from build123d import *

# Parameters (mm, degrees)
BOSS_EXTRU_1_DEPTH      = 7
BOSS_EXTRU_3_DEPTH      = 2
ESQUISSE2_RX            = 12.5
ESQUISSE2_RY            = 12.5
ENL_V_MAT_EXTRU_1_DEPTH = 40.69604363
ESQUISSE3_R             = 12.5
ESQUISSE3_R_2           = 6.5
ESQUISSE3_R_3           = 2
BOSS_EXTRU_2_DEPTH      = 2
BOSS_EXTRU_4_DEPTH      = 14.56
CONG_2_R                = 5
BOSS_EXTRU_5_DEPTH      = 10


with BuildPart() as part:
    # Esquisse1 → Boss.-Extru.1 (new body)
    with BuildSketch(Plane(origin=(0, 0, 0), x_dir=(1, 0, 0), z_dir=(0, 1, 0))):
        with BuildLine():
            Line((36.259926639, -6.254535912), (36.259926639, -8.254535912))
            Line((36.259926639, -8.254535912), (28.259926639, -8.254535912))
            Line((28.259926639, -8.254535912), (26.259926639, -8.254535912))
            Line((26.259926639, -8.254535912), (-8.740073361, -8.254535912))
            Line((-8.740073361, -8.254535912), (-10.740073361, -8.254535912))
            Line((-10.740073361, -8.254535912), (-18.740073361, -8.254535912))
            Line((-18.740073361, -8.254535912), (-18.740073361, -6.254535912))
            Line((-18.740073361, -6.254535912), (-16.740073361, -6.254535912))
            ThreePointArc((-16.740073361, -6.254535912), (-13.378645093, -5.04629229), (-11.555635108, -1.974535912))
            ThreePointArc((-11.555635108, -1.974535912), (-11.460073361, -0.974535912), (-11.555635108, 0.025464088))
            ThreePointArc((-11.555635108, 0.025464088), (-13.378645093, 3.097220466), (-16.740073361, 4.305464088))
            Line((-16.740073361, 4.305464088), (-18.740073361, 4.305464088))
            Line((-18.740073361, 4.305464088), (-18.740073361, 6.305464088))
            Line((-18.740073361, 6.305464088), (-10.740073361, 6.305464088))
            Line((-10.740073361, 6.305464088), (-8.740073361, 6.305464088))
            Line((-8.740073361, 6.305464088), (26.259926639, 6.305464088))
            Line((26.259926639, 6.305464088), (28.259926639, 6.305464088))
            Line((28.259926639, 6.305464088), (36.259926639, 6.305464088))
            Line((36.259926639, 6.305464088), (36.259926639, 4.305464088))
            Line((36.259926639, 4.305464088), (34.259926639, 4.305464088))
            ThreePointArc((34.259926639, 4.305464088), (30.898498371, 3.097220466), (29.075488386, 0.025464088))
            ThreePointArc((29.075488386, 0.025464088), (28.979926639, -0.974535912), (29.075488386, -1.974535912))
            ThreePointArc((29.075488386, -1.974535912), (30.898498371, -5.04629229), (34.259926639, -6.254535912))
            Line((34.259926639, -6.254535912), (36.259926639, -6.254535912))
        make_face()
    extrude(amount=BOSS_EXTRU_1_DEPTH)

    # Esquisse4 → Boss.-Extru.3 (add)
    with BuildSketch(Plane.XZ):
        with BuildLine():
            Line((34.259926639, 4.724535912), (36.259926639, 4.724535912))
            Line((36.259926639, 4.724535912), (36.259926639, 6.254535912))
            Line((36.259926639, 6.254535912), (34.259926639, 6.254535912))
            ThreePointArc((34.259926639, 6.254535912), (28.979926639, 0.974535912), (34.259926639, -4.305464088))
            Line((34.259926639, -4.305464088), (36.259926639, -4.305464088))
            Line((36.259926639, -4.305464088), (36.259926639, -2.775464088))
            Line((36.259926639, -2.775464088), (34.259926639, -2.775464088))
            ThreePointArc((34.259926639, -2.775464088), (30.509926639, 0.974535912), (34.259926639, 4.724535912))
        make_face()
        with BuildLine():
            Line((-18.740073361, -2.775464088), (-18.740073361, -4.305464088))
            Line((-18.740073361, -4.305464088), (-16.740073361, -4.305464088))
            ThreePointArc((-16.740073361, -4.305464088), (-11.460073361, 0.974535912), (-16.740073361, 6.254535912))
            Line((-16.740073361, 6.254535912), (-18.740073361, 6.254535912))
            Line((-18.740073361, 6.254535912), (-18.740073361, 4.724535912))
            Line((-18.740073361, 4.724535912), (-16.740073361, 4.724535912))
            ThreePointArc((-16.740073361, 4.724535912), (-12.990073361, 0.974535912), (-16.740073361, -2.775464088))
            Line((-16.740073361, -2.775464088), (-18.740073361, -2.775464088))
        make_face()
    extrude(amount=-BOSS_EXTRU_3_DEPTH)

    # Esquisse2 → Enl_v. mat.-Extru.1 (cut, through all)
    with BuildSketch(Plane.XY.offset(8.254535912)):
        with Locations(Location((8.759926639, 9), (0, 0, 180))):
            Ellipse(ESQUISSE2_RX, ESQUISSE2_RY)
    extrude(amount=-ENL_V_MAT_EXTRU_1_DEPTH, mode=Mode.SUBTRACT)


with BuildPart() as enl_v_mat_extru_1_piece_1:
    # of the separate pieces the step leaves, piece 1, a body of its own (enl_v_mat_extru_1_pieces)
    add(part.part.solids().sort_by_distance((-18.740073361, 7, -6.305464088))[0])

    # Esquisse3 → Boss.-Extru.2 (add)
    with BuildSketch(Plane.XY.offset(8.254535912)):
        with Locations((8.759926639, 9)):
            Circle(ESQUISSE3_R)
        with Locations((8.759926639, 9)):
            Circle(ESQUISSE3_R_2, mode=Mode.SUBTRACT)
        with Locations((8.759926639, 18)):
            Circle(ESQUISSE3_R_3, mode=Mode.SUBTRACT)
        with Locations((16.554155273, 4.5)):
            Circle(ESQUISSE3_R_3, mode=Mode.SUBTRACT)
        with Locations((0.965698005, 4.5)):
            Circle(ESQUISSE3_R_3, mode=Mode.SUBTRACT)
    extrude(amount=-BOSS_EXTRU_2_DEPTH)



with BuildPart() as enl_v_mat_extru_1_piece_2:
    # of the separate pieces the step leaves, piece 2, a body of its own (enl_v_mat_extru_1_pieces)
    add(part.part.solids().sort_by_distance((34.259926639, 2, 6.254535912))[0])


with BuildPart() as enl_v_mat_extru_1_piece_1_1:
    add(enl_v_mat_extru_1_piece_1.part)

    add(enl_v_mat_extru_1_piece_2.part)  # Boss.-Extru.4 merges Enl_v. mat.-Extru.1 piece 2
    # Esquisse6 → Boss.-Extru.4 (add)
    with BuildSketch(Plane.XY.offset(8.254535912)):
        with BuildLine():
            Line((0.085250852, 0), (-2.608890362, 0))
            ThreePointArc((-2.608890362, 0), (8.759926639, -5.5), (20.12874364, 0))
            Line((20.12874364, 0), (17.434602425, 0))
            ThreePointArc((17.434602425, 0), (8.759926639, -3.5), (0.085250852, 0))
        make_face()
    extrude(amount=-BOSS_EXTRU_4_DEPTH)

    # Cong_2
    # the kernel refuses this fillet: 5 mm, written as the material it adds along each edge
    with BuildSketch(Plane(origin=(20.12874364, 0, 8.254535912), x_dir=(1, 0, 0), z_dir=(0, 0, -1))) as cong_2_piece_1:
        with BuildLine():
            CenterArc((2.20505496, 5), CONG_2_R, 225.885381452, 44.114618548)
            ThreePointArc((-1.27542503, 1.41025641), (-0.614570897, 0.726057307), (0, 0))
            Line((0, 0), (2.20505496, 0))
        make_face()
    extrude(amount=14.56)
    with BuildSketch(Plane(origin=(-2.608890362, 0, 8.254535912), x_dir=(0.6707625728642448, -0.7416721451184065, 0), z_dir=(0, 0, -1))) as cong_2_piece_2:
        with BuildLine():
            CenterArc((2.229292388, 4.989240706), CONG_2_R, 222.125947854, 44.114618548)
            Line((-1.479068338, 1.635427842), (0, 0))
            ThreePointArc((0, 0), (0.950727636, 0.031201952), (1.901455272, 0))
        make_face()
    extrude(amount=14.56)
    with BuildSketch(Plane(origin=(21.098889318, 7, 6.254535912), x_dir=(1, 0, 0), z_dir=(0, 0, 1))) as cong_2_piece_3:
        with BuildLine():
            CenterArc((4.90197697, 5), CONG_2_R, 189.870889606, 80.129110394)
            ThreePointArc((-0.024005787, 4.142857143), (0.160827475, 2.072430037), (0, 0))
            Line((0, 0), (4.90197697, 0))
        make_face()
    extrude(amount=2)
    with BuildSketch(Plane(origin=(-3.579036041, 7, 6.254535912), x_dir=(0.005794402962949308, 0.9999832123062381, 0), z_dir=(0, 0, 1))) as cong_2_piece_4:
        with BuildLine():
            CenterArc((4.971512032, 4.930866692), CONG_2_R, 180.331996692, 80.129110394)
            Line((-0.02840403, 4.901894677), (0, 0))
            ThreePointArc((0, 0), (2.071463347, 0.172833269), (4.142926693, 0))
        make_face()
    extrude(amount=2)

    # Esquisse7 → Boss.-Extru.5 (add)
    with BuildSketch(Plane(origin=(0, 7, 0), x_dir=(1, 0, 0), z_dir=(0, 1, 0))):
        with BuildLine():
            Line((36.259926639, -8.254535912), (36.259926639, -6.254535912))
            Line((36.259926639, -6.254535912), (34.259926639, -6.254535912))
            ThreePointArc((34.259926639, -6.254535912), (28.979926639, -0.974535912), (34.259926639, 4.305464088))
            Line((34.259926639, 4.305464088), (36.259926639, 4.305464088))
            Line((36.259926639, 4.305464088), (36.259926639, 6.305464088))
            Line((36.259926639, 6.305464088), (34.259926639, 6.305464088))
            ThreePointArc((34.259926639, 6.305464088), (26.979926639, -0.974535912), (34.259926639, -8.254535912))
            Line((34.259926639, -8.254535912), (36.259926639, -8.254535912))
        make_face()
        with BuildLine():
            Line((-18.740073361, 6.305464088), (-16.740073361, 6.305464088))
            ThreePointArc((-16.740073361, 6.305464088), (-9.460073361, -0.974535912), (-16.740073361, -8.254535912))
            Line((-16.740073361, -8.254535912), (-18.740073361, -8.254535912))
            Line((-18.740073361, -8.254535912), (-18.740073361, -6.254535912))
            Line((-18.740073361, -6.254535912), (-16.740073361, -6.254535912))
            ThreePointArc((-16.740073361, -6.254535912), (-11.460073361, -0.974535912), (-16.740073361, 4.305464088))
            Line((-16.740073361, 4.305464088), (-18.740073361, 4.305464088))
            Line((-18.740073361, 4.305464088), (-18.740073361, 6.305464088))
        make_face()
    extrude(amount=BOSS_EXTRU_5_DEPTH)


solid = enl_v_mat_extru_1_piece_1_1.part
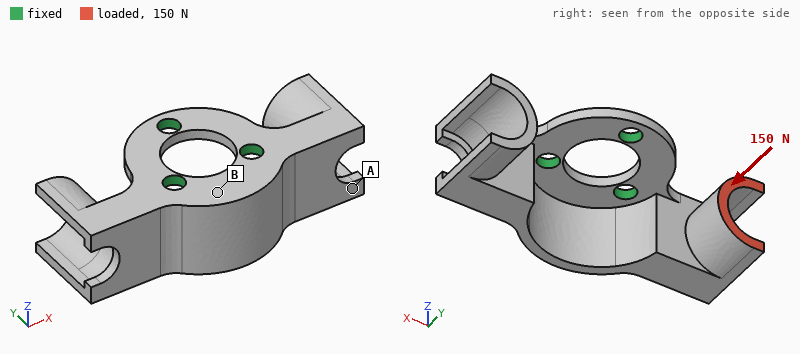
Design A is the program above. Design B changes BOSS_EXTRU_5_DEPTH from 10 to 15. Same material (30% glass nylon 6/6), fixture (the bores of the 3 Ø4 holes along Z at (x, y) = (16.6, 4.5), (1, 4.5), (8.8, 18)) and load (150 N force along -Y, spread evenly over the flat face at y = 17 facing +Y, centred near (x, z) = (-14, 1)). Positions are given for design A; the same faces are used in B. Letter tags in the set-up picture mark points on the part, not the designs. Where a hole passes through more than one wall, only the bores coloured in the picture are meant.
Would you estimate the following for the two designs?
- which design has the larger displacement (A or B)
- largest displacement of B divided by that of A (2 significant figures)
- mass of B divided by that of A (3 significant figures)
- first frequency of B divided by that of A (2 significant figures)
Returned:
B
1.1
1.10
0.92
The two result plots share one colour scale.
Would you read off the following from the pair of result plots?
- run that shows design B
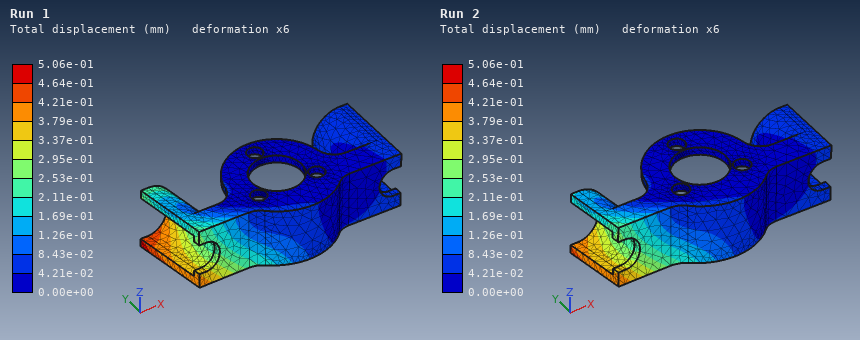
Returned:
Run 1
